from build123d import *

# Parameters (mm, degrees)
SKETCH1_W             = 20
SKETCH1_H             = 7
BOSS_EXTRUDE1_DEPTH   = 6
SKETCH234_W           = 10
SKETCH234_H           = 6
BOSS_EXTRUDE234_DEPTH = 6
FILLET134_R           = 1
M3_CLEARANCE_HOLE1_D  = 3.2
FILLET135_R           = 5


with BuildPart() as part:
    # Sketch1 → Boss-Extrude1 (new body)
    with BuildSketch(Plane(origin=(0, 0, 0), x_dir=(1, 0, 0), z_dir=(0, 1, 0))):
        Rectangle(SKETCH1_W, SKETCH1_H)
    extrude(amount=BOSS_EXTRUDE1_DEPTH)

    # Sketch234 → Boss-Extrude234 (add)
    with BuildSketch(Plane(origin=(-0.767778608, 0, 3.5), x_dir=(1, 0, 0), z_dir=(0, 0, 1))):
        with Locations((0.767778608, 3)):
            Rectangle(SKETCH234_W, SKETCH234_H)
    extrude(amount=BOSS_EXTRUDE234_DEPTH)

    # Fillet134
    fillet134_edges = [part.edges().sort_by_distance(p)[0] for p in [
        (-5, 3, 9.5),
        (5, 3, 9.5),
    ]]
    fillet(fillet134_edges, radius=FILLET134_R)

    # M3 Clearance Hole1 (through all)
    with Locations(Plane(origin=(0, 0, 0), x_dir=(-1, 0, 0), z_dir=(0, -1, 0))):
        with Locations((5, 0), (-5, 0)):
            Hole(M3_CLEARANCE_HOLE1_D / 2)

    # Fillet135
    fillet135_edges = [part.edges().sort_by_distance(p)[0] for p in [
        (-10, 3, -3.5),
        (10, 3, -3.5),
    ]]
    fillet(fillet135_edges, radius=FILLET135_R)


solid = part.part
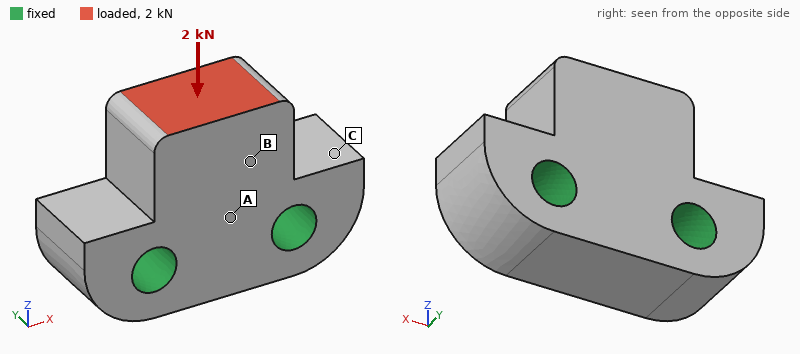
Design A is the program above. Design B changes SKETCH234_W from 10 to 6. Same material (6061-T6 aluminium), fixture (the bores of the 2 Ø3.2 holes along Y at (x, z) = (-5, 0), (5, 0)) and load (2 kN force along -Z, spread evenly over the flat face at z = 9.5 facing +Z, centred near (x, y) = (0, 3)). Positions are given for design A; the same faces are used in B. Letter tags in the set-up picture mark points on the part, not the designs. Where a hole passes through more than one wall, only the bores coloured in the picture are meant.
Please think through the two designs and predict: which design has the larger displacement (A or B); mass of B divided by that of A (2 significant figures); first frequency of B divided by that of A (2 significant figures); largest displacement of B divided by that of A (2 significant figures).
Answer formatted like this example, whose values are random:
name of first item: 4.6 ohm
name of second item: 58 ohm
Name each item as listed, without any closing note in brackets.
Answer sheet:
which design has the larger displacement: B
mass of B divided by that of A: 0.86
first frequency of B divided by that of A: 0.97
largest displacement of B divided by that of A: 1.8
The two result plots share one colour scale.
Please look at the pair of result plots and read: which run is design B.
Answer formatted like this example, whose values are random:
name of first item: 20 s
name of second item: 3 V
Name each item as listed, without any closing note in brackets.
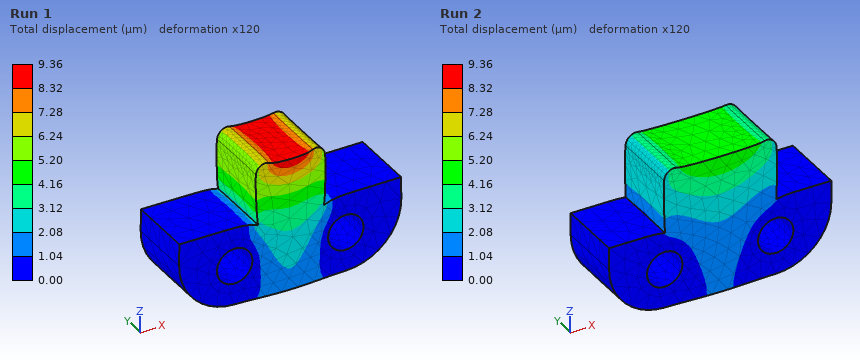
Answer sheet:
which run is design B: Run 1
